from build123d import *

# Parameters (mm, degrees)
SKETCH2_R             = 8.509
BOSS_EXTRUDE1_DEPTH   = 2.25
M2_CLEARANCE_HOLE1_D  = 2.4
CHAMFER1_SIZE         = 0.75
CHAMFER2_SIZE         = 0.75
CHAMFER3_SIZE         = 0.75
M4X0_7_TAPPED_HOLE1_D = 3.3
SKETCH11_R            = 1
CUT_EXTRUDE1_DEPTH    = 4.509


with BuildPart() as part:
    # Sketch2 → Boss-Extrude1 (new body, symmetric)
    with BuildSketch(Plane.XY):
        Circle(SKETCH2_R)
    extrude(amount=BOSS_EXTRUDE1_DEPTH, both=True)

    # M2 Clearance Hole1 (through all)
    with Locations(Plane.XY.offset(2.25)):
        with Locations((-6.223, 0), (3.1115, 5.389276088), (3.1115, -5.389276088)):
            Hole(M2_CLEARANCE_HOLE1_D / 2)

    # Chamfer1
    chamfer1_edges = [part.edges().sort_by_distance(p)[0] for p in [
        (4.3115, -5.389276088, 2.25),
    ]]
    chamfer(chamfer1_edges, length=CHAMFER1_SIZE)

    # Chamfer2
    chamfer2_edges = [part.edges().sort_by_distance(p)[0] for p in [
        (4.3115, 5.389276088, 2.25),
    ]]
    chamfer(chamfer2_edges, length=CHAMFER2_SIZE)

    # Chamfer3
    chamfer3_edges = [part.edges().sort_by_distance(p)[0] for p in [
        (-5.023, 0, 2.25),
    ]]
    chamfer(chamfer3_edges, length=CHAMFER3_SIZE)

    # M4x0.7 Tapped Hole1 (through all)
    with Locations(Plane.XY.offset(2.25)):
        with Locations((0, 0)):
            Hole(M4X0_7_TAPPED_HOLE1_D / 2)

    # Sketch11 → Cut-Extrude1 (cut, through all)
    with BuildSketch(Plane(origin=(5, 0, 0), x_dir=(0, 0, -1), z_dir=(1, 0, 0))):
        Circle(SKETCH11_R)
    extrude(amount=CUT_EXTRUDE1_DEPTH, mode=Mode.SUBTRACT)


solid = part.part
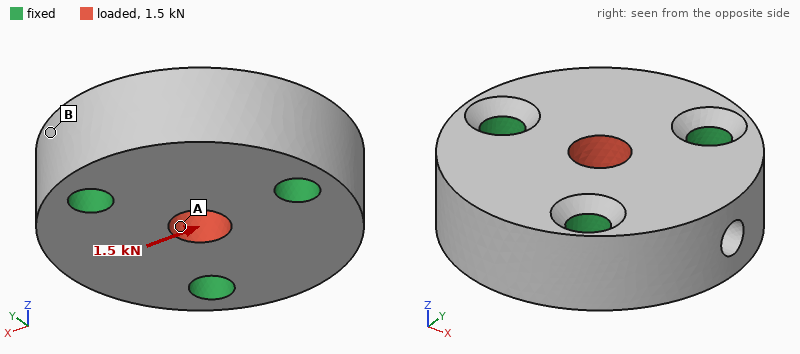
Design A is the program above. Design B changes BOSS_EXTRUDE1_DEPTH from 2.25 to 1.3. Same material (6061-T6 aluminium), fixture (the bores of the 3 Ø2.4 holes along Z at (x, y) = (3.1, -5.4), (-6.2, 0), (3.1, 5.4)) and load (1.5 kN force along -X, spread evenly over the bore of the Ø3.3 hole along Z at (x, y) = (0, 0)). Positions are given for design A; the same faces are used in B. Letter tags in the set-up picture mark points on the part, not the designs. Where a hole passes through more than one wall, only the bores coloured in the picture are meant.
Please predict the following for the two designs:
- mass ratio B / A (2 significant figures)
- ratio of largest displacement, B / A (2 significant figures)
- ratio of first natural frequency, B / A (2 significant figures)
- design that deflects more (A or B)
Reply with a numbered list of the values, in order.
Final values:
1. 0.57
2. 1.8
3. 0.71
4. B
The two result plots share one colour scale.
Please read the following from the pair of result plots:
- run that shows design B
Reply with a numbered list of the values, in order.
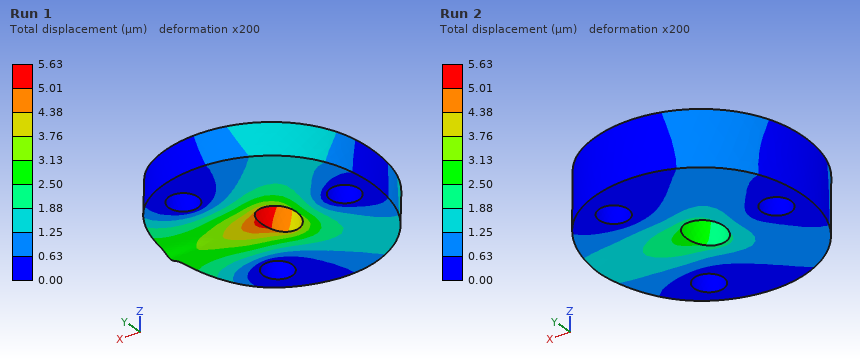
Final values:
1. Run 1
